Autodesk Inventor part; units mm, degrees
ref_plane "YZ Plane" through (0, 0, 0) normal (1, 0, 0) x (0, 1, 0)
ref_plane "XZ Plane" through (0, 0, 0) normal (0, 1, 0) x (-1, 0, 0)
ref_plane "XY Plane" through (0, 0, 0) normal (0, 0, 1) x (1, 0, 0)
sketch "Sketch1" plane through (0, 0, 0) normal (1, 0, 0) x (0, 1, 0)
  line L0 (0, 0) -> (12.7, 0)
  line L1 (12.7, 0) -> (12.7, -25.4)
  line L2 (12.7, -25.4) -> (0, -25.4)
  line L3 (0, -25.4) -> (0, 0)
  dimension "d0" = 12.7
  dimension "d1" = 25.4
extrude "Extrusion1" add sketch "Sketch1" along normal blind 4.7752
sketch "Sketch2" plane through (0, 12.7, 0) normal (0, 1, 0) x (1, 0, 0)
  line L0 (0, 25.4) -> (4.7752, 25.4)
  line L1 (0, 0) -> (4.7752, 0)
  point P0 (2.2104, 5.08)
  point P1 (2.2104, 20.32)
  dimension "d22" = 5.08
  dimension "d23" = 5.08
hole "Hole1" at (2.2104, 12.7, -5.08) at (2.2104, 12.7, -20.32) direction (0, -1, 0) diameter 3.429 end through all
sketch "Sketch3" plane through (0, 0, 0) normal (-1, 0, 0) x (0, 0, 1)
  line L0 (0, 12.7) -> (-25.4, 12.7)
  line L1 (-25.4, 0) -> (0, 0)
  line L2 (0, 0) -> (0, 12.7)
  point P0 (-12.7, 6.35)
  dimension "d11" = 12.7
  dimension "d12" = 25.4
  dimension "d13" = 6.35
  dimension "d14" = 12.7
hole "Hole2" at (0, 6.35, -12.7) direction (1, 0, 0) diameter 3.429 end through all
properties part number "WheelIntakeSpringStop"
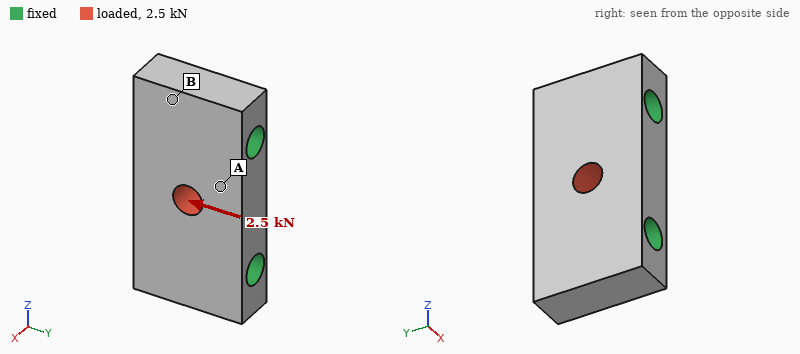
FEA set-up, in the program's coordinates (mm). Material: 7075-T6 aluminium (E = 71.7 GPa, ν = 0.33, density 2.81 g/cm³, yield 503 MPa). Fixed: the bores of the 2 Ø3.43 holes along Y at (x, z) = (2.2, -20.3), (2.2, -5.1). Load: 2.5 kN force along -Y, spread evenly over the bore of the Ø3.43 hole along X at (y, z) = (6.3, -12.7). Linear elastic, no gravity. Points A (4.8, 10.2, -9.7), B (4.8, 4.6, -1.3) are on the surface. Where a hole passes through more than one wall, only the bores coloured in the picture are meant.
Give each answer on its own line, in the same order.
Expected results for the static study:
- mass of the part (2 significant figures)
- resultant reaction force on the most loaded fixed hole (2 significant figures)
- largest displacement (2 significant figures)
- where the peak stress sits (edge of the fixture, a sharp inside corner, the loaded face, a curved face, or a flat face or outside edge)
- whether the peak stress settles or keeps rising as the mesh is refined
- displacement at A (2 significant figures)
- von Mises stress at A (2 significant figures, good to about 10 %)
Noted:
3.5 g
1.3 kN
5.8 µm
edge of the fixture
keeps rising
3.0 µm
39 MPa
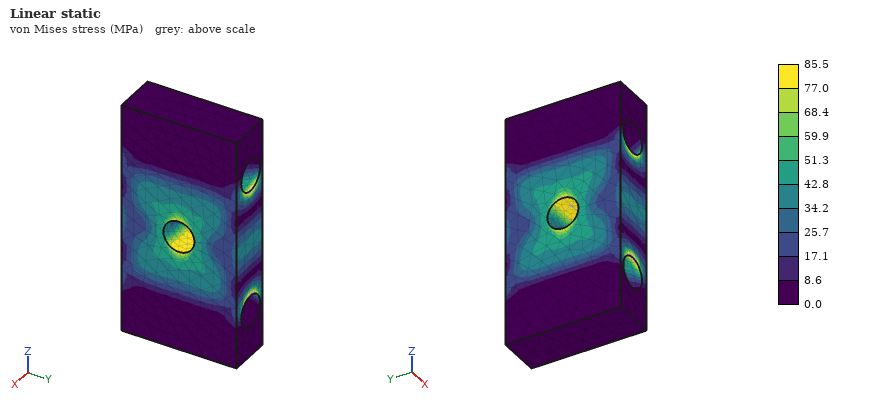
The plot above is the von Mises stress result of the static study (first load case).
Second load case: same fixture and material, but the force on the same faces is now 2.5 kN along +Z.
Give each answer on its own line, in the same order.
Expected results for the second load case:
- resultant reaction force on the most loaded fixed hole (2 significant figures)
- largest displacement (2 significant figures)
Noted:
1.3 kN
2.8 µm
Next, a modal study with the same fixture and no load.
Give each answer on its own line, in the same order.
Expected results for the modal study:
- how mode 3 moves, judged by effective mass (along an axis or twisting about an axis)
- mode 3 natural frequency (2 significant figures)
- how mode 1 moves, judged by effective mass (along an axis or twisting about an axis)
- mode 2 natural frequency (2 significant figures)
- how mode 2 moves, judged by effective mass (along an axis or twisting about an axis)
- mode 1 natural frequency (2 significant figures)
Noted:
along Y
120 kHz
along X
98 kHz
twisting about Z
89 kHz
